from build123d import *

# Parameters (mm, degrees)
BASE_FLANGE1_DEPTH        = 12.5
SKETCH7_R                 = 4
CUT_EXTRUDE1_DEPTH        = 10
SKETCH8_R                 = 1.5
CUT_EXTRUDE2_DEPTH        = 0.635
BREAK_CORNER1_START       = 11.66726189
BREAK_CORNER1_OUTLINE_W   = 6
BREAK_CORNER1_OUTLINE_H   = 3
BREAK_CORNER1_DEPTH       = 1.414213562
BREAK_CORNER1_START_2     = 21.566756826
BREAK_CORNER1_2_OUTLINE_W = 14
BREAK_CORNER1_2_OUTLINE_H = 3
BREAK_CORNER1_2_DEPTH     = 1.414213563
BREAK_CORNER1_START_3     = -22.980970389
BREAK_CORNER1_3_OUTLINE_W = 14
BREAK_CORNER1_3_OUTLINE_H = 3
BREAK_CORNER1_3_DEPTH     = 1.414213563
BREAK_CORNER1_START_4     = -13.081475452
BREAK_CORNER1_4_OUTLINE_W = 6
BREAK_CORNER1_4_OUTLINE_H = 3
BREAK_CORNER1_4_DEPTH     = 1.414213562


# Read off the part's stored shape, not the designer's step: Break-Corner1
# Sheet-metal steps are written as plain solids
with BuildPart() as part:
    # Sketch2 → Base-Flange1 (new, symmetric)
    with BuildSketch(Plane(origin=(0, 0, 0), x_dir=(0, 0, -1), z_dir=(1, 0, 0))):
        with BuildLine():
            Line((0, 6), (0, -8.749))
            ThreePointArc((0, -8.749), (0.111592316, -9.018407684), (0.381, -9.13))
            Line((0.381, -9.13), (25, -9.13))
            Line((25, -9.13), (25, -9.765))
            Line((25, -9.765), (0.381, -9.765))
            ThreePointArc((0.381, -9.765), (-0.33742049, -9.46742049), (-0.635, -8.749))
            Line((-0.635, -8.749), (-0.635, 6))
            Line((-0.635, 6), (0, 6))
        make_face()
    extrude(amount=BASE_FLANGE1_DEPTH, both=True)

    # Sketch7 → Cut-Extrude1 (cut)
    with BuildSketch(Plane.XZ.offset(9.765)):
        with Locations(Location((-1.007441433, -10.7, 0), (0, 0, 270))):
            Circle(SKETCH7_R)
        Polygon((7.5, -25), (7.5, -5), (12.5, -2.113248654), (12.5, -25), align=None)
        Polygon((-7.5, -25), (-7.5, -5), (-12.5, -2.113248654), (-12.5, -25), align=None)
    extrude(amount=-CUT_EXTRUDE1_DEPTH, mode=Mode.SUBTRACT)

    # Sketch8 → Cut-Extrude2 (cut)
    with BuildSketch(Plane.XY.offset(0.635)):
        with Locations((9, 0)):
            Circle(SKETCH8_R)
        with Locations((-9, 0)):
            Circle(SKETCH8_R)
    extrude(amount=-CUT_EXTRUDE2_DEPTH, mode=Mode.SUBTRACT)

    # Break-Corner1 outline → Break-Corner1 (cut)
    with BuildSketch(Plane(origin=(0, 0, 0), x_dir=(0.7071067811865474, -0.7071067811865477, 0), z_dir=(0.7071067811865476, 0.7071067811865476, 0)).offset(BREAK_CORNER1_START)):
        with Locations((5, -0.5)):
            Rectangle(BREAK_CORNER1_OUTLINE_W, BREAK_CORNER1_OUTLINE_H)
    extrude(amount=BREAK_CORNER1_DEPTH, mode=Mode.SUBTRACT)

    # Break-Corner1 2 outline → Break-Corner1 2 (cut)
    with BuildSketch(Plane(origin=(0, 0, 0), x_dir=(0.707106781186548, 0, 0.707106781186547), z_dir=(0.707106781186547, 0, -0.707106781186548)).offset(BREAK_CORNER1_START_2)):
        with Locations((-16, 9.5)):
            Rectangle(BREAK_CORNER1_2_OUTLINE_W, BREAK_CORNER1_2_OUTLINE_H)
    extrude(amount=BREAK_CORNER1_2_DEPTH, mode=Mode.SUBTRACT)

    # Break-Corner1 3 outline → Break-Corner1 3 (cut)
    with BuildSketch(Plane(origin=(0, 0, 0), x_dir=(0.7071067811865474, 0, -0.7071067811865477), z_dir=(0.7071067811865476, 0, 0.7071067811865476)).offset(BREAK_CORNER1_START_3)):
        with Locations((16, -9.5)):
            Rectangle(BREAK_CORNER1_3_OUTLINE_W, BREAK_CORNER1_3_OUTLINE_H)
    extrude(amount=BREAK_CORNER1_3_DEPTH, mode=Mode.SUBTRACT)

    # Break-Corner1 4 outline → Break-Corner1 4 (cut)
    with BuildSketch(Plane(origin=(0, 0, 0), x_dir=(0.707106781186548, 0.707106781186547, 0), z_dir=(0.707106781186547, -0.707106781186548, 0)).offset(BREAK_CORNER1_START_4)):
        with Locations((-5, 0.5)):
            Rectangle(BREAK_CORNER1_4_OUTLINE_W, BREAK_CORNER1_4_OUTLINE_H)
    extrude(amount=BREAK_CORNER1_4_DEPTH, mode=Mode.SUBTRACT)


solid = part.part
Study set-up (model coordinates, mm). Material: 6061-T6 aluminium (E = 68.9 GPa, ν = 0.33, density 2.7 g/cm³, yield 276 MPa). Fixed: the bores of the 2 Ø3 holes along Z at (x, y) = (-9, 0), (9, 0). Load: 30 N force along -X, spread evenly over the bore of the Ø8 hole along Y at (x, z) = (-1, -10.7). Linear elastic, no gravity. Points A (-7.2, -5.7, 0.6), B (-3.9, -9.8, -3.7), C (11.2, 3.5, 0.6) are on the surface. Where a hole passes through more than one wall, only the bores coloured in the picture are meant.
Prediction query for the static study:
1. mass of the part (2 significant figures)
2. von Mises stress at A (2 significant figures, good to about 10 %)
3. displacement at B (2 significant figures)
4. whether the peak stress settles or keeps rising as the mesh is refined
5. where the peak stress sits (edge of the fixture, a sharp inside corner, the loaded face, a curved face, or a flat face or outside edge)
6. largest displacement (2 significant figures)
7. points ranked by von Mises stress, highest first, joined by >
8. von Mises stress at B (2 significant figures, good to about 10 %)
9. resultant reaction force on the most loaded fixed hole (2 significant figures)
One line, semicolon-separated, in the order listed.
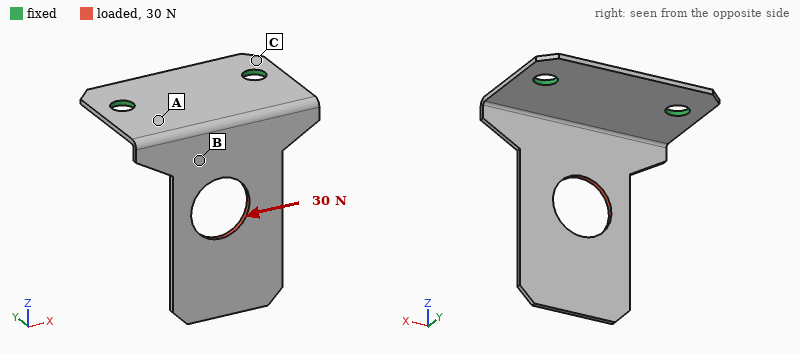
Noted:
1.2 g; 66 MPa; 0.083 mm; keeps rising; edge of the fixture; 0.38 mm; A > B > C; 37 MPa; 27 N
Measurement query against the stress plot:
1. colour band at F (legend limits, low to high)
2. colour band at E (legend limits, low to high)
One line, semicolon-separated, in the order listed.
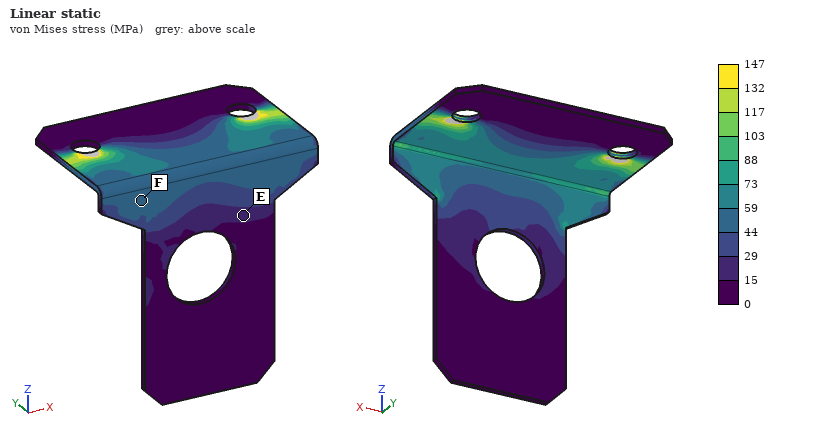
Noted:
44 to 59 MPa; 15 to 29 MPa
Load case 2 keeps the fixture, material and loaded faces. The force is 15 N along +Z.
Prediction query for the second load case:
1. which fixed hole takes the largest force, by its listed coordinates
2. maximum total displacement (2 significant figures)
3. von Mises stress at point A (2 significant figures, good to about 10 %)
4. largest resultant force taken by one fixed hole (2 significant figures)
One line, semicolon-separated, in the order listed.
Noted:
(-9, 0); 0.39 mm; 34 MPa; 8.3 N
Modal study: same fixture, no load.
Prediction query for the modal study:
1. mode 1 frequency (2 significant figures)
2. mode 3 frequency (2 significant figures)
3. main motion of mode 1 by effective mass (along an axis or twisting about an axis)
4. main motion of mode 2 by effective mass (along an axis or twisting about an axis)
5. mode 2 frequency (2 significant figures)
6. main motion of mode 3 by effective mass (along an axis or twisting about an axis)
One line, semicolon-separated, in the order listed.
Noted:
620 Hz; 2600 Hz; along Y; along X; 1900 Hz; along Z
